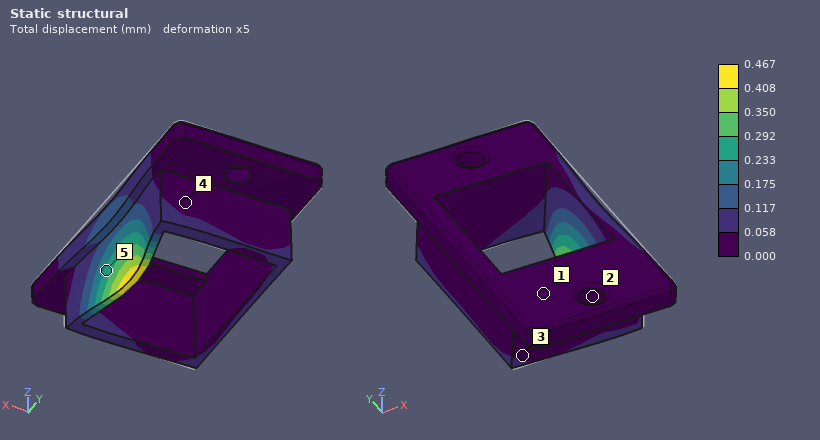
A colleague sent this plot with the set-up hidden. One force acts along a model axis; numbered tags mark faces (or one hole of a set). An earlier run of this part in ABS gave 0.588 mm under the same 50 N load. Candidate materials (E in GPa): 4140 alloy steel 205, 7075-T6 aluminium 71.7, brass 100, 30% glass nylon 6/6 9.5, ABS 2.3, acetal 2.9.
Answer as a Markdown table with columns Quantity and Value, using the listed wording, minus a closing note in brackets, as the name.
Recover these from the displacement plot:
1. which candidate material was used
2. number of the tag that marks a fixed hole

| Quantity | Value |
|---|---|
| which candidate material was used | acetal |
| number of the tag that marks a fixed hole | 2 |
